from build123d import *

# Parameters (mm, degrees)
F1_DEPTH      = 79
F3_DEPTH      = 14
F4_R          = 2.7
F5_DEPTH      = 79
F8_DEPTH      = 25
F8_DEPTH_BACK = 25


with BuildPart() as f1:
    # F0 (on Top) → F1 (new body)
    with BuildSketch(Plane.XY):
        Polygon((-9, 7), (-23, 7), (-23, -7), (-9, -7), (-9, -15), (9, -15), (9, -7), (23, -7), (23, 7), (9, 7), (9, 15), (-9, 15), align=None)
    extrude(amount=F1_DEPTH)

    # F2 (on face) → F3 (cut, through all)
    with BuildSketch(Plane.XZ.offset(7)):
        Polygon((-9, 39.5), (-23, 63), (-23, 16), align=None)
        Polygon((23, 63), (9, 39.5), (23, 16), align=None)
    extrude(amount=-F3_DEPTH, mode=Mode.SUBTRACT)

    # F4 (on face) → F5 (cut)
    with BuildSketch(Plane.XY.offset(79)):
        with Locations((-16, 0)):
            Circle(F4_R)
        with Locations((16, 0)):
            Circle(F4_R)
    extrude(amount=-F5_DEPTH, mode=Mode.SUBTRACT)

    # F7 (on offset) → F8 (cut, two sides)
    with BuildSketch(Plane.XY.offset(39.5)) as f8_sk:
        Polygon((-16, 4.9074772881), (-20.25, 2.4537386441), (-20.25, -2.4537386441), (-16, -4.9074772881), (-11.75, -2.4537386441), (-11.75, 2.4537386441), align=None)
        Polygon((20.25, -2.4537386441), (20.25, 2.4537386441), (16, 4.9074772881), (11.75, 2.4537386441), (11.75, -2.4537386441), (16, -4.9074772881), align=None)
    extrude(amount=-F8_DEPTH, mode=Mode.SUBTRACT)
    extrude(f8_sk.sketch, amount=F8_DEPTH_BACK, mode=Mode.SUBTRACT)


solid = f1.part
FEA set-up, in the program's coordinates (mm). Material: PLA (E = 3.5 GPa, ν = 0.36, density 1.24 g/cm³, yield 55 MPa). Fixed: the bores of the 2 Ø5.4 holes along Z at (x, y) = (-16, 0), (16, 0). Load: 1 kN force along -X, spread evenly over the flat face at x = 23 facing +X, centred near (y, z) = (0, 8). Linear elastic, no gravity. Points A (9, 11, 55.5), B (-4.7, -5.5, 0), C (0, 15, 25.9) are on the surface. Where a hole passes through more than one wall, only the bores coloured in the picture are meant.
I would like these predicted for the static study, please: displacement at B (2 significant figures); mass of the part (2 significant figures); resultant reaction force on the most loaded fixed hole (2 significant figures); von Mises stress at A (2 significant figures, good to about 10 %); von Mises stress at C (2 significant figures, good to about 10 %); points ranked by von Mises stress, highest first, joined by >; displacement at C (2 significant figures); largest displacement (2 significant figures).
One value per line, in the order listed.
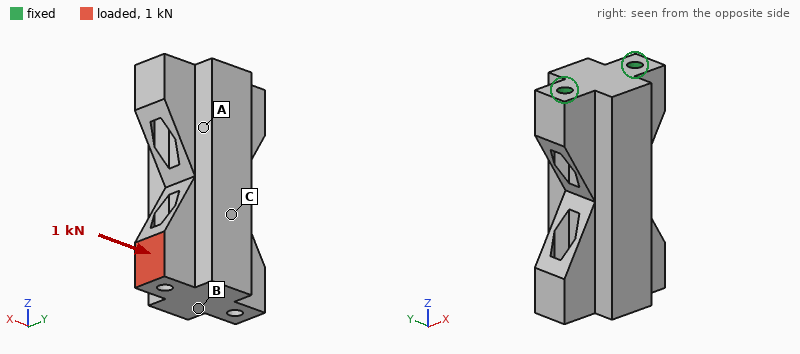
0.96 mm
74 g
1.9 kN
11 MPa
5.6 MPa
A > C > B
0.43 mm
1.1 mm
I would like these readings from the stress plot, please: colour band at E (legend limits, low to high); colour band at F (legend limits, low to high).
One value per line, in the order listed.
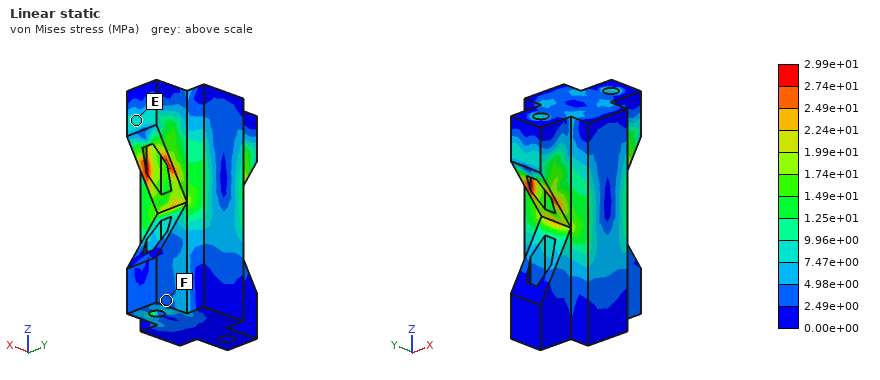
7.47e+00 to 9.96e+00 MPa
2.49e+00 to 4.98e+00 MPa
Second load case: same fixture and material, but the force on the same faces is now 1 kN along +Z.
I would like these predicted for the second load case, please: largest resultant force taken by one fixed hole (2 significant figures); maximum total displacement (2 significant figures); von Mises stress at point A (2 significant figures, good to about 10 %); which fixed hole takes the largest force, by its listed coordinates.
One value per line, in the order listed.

1.2 kN
0.74 mm
7.1 MPa
(16, 0)
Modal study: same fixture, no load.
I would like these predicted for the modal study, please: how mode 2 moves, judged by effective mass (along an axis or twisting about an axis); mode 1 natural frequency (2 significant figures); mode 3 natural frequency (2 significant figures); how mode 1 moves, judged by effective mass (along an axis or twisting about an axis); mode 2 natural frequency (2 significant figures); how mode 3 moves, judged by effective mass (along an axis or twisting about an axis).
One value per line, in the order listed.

along X
670 Hz
2500 Hz
along Y
1100 Hz
twisting about Z
